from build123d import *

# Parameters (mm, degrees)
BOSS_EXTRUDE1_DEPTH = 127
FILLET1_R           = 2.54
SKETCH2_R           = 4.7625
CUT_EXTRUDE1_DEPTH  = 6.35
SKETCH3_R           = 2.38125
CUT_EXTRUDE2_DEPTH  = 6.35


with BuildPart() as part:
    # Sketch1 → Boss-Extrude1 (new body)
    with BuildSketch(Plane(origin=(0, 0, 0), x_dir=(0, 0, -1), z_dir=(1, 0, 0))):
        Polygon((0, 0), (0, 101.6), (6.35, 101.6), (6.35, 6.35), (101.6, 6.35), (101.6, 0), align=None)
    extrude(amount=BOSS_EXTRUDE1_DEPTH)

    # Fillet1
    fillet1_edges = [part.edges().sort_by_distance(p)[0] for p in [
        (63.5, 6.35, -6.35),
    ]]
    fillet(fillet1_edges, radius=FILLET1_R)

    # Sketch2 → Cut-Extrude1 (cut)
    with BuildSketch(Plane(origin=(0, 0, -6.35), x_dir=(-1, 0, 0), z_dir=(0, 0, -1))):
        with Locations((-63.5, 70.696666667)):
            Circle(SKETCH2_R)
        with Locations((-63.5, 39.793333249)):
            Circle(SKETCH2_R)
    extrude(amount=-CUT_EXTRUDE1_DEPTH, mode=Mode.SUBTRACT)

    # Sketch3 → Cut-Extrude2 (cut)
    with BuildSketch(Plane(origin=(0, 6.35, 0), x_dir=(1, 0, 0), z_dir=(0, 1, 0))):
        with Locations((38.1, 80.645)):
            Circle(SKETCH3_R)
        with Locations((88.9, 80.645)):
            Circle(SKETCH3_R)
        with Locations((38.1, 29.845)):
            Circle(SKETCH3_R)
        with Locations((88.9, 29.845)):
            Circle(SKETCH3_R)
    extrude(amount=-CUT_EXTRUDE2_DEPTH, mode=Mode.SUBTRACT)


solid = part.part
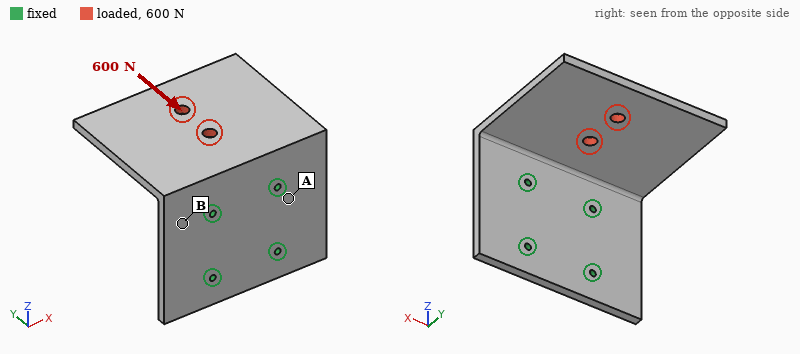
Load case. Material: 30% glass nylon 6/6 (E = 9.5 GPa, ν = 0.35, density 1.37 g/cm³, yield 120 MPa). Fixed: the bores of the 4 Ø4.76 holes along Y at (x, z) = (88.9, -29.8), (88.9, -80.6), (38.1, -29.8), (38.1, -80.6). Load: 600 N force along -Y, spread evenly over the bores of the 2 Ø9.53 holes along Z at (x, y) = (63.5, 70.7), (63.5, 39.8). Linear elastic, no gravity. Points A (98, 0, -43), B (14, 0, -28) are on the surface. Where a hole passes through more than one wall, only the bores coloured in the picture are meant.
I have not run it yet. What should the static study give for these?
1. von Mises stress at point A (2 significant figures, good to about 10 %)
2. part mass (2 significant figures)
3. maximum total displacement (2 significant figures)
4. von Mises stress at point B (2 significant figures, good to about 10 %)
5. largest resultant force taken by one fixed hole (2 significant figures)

3.7 MPa
220 g
1.1 mm
8.2 MPa
370 N
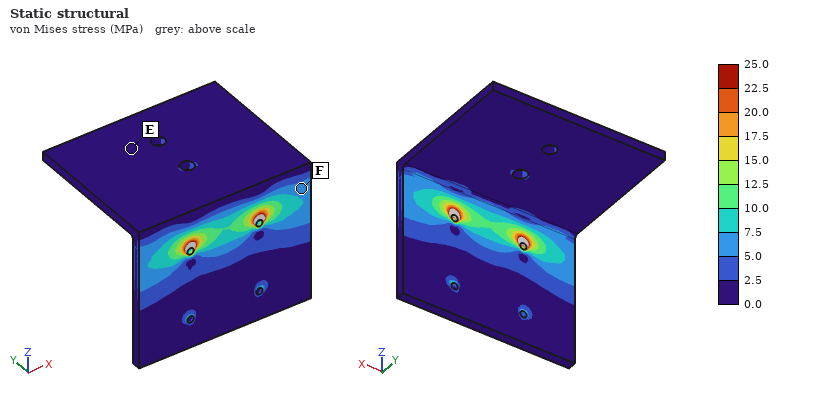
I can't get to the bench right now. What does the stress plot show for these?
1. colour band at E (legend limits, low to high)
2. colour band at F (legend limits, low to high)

0.0 to 2.5 MPa
5.0 to 7.5 MPa
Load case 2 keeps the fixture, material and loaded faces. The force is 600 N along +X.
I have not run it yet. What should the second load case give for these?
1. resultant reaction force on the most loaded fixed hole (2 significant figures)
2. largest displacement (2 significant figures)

670 N
0.90 mm
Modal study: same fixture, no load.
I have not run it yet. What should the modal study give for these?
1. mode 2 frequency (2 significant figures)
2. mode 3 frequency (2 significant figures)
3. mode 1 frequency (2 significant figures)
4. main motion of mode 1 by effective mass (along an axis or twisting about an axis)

410 Hz
600 Hz
200 Hz
along Z
